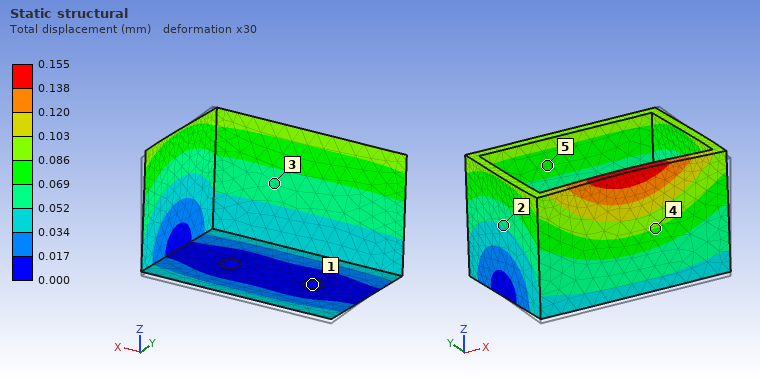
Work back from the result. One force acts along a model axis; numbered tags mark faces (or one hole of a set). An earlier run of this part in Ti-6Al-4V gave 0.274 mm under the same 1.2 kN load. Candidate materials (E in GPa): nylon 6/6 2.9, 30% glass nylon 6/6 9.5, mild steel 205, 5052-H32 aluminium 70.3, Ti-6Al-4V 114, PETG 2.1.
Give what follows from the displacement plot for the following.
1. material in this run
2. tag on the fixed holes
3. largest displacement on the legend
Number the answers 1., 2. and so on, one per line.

1. mild steel
2. 1
3. 0.155 mm
